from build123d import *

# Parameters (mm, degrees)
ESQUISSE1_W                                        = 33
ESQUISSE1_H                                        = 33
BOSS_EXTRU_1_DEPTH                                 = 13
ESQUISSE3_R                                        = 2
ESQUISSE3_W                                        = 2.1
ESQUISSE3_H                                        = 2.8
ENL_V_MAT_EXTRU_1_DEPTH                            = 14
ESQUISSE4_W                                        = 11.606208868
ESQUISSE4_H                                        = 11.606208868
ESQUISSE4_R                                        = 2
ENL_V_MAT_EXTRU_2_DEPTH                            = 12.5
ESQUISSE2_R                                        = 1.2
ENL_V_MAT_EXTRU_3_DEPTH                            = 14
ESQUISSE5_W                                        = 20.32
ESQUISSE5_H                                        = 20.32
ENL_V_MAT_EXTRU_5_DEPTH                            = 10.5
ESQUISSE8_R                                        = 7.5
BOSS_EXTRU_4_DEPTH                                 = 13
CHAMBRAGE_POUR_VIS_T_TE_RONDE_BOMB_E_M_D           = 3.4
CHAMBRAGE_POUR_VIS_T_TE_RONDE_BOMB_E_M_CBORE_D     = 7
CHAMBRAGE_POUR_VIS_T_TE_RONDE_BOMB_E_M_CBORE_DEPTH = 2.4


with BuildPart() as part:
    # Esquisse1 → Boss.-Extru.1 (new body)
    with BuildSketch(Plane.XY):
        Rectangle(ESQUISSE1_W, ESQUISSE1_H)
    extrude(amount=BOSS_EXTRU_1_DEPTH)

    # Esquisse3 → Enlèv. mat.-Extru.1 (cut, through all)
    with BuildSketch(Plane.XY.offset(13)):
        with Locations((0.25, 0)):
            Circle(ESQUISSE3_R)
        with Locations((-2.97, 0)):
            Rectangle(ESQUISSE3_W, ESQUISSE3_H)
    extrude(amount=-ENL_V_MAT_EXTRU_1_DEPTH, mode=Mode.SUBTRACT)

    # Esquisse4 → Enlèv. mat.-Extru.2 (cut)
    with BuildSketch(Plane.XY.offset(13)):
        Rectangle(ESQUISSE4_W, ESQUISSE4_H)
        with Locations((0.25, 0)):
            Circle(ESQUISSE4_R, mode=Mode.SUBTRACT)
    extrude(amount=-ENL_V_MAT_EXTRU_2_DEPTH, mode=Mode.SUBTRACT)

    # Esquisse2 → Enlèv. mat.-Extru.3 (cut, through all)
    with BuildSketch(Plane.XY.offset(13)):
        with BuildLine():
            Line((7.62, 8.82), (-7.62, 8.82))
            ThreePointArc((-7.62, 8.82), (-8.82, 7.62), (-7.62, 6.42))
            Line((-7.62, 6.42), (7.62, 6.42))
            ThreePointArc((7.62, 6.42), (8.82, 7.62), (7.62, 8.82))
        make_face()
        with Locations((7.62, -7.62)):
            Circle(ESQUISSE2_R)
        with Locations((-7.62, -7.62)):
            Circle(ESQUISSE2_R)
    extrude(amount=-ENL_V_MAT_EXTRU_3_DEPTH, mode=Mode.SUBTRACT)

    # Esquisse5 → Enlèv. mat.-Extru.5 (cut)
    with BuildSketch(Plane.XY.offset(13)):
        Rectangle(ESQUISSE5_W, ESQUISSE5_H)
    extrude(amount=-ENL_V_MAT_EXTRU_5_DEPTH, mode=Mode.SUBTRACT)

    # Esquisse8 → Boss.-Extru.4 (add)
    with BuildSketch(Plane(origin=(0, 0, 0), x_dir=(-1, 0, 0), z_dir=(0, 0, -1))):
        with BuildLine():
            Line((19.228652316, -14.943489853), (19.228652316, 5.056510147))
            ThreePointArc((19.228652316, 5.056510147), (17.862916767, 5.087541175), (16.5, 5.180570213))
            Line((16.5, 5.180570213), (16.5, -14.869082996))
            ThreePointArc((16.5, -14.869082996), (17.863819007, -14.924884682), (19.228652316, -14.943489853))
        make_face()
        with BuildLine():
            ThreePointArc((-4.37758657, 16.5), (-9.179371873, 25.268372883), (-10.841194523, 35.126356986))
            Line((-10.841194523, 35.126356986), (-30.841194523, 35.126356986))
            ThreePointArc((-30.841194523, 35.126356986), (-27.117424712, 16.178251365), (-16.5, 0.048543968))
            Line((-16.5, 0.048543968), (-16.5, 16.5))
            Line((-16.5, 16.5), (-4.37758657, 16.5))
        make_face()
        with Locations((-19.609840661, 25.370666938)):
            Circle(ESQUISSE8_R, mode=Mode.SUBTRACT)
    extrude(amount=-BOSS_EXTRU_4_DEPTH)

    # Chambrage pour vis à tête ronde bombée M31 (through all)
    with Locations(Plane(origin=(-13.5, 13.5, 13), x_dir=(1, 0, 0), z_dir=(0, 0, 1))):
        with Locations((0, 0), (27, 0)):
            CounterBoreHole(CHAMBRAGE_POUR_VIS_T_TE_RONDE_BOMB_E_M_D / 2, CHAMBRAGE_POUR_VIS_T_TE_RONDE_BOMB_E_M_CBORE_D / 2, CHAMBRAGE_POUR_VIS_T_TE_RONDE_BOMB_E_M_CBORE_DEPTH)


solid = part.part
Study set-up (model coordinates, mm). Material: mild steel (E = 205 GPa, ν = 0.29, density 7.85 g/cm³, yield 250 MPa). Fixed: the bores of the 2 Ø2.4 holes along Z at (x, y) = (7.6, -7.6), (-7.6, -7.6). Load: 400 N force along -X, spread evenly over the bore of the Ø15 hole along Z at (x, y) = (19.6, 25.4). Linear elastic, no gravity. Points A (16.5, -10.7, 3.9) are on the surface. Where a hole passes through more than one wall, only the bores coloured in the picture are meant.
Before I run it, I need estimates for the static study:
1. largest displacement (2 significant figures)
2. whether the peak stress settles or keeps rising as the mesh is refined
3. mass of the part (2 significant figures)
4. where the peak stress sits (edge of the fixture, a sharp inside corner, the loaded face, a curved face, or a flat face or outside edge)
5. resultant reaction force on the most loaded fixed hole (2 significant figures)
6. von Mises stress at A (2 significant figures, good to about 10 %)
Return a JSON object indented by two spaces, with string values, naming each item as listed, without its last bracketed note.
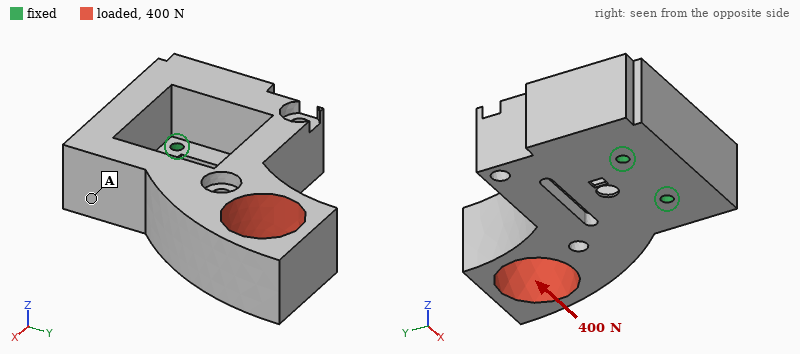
{
  "largest displacement": "26 µm",
  "whether the peak stress settles or keeps rising as the mesh is refined": "keeps rising",
  "mass of the part": "110 g",
  "where the peak stress sits": "edge of the fixture",
  "resultant reaction force on the most loaded fixed hole": "790 N",
  "von Mises stress at A": "10 MPa"
}
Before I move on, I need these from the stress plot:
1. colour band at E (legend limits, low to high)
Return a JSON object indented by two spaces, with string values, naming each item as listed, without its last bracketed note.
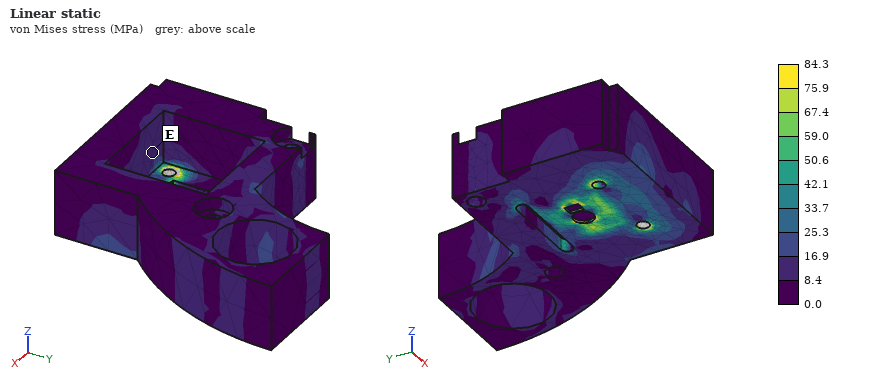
{
  "colour band at E": "8.4 to 16.9 MPa"
}
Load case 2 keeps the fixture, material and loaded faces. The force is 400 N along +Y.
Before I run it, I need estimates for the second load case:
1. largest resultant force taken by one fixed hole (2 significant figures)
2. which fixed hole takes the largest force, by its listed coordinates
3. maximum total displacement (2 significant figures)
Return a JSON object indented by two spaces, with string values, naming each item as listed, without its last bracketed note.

{
  "largest resultant force taken by one fixed hole": "660 N",
  "which fixed hole takes the largest force, by its listed coordinates": "(7.6, -7.6)",
  "maximum total displacement": "28 µm"
}
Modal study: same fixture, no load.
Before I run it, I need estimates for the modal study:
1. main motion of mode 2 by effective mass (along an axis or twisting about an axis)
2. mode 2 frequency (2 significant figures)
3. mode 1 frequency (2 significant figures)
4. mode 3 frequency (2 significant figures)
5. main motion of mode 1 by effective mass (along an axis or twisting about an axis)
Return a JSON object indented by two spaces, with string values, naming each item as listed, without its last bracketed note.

{
  "main motion of mode 2 by effective mass": "along X",
  "mode 2 frequency": "3700 Hz",
  "mode 1 frequency": "1400 Hz",
  "mode 3 frequency": "6000 Hz",
  "main motion of mode 1 by effective mass": "along Z"
}
